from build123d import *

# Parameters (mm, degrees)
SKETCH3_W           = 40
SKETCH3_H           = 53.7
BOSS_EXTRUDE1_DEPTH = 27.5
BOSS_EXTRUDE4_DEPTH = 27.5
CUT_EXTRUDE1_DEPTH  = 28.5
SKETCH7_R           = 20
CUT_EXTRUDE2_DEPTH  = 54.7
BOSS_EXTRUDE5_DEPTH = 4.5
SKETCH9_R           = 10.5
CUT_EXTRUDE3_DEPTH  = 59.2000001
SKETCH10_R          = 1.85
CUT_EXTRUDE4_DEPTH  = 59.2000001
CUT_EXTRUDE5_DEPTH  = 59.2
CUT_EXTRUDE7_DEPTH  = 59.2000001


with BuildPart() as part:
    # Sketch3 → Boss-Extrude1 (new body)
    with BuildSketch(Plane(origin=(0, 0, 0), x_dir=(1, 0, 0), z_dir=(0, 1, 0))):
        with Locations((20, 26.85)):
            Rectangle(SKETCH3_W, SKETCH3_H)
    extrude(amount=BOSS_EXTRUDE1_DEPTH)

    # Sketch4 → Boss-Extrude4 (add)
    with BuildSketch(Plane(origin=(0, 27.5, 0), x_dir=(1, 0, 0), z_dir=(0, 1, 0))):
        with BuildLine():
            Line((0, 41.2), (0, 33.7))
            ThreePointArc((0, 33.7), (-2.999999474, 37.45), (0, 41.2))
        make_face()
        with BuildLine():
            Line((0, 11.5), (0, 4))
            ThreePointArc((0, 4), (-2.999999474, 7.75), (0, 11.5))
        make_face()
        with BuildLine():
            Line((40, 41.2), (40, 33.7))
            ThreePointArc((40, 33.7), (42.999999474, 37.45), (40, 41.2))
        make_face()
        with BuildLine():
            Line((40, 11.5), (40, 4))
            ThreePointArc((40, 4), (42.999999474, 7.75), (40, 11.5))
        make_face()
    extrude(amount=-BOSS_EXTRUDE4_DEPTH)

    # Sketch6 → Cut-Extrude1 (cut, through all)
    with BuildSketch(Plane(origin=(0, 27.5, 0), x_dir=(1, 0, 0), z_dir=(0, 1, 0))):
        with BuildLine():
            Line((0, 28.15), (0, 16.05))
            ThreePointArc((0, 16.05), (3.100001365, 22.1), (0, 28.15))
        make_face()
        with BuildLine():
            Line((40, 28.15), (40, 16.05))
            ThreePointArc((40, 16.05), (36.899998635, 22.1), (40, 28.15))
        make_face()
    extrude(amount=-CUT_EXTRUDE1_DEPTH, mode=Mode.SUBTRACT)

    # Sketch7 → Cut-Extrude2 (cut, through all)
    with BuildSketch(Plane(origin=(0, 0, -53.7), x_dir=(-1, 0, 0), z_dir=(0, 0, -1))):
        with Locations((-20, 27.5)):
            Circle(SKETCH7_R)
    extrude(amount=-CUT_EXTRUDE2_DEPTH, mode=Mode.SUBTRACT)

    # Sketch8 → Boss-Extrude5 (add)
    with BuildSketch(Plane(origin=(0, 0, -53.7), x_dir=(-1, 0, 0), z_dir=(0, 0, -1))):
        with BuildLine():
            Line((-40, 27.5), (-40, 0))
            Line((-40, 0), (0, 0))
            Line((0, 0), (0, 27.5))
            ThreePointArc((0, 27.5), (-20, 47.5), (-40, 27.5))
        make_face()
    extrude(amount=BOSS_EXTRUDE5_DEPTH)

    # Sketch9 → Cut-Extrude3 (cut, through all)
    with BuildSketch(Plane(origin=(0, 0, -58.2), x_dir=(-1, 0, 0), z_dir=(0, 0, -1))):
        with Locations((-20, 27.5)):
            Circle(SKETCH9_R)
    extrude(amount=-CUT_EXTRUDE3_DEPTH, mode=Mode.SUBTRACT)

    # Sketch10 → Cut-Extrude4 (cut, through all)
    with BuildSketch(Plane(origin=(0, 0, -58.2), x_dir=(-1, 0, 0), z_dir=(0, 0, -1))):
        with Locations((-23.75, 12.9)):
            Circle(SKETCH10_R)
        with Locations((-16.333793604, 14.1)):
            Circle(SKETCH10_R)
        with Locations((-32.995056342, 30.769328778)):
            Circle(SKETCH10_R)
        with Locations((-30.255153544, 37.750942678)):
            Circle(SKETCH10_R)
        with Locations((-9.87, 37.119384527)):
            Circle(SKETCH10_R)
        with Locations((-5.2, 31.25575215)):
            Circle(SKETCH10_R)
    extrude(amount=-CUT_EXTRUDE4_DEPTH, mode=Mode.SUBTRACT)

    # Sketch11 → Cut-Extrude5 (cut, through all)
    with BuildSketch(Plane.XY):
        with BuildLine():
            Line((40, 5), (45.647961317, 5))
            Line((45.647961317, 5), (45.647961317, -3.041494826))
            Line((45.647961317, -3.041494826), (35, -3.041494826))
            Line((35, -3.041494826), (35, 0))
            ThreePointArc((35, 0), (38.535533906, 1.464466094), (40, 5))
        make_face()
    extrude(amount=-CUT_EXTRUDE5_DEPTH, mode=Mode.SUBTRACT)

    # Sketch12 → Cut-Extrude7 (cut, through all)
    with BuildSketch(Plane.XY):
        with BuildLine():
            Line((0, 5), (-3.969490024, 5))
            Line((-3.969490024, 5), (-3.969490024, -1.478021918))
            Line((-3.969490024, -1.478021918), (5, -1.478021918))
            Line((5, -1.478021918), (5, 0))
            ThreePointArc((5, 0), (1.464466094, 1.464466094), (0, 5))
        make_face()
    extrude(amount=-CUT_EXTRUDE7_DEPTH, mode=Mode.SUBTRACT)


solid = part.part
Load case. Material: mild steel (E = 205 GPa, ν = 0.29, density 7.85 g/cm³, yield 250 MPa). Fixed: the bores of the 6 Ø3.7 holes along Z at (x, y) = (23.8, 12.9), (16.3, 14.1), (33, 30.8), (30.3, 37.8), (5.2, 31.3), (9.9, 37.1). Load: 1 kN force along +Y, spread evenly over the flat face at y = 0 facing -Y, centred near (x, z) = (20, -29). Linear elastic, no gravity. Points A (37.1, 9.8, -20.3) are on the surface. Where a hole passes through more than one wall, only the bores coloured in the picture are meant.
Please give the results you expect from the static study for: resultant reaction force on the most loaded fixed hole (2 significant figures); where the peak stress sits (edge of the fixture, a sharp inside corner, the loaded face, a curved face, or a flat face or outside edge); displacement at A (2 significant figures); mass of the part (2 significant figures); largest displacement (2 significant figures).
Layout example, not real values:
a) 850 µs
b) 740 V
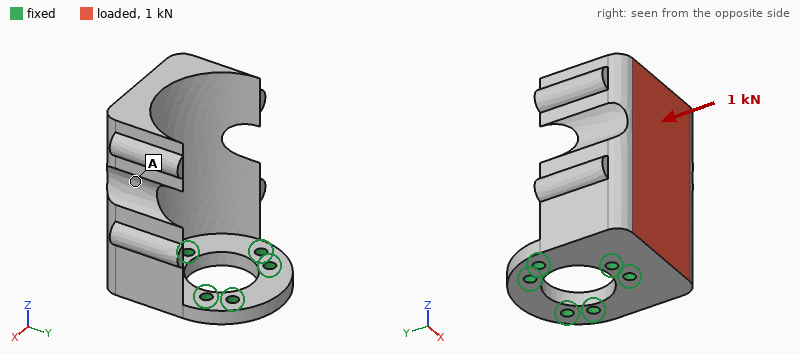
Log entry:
a) 810 N
b) a curved face
c) 41 µm
d) 240 g
e) 69 µm
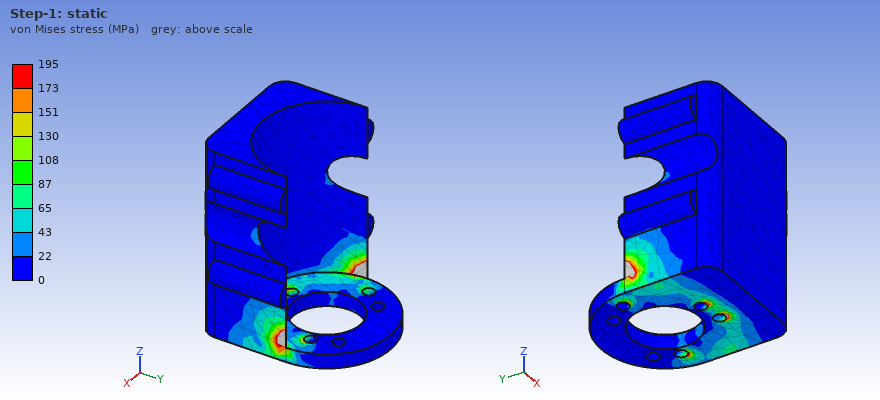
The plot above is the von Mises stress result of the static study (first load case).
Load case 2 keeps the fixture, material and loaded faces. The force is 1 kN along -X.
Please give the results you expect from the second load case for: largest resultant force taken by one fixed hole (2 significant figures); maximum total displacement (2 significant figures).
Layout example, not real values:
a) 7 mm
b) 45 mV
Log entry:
a) 1.1 kN
b) 40 µm
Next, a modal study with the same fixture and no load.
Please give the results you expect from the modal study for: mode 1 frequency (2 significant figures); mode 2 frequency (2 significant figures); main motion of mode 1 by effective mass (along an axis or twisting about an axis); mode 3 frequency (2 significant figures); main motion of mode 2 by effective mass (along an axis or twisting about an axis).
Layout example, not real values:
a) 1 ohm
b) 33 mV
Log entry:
a) 1600 Hz
b) 2000 Hz
c) along Y
d) 5200 Hz
e) along X
